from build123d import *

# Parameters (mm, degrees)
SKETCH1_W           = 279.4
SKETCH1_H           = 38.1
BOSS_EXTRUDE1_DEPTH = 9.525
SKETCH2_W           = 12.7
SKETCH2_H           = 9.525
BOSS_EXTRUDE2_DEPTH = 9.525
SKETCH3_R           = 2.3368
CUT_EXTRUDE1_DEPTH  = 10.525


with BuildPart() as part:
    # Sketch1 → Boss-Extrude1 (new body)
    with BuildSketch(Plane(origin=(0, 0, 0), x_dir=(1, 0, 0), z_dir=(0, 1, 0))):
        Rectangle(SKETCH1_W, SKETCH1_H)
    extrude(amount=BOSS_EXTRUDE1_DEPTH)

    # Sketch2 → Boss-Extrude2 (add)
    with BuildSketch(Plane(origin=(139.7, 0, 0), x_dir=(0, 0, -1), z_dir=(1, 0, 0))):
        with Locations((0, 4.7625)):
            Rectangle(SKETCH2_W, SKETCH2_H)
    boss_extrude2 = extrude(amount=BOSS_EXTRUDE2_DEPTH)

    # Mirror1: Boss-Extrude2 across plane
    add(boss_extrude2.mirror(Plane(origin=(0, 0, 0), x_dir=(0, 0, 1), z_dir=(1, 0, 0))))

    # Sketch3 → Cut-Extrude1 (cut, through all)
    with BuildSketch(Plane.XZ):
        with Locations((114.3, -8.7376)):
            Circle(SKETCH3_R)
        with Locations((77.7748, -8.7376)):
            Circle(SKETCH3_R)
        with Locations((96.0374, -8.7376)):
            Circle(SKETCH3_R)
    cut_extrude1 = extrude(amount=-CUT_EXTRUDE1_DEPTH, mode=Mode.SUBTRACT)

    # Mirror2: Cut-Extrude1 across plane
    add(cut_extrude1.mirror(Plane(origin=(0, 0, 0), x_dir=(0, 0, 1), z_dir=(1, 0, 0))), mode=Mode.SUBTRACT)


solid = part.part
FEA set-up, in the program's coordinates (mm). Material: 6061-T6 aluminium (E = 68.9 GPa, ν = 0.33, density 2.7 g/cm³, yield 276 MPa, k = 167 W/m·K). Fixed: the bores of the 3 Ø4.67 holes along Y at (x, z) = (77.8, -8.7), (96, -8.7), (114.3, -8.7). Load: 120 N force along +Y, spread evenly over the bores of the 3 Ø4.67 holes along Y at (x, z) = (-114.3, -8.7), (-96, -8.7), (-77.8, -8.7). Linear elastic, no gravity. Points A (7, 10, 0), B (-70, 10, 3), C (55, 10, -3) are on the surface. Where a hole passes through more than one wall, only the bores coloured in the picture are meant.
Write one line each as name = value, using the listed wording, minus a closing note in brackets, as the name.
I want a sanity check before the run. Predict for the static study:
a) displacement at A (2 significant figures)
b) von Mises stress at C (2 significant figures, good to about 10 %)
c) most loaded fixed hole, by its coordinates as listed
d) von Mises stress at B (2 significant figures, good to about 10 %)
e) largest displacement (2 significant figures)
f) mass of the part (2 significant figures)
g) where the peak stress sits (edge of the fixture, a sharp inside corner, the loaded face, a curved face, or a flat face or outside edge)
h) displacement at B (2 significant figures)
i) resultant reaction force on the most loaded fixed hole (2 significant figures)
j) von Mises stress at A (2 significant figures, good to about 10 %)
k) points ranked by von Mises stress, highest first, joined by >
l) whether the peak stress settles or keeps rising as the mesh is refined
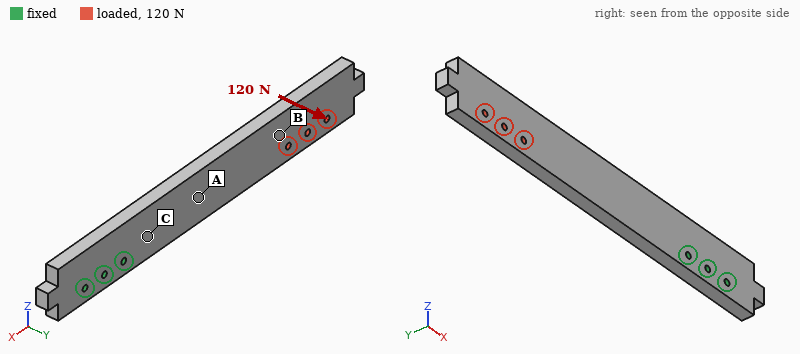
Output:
displacement at A = 0.26 mm
von Mises stress at C = 31 MPa
most loaded fixed hole, by its coordinates as listed = (77.8, -8.7)
von Mises stress at B = 5.9 MPa
largest displacement = 1.7 mm
mass of the part = 280 g
where the peak stress sits = edge of the fixture
displacement at B = 0.91 mm
resultant reaction force on the most loaded fixed hole = 590 N
von Mises stress at A = 22 MPa
points ranked by von Mises stress, highest first, joined by > = C > A > B
whether the peak stress settles or keeps rising as the mesh is refined = keeps rising
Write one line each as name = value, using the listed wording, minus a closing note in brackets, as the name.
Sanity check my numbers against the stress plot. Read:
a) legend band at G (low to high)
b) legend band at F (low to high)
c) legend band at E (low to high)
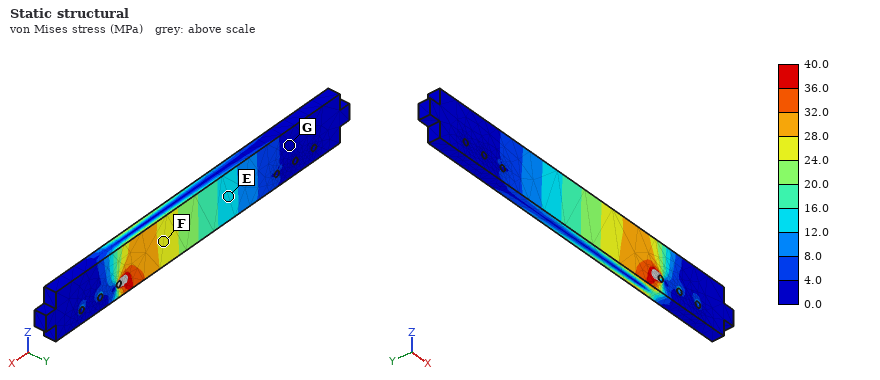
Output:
legend band at G = 0.0 to 4.0 MPa
legend band at F = 24.0 to 28.0 MPa
legend band at E = 12.0 to 16.0 MPa
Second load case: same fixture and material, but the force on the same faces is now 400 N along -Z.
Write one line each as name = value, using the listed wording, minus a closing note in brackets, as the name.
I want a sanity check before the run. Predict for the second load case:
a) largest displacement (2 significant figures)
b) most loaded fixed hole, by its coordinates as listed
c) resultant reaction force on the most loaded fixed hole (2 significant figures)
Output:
largest displacement = 0.45 mm
most loaded fixed hole, by its coordinates as listed = (77.8, -8.7)
resultant reaction force on the most loaded fixed hole = 2.7 kN
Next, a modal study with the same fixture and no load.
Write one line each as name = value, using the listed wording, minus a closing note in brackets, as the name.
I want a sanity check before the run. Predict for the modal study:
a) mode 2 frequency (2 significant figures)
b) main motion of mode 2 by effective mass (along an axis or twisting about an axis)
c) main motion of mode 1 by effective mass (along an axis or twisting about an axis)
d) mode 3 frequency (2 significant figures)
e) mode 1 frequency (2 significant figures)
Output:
mode 2 frequency = 540 Hz
main motion of mode 2 by effective mass = along Z
main motion of mode 1 by effective mass = along Y
mode 3 frequency = 960 Hz
mode 1 frequency = 160 Hz
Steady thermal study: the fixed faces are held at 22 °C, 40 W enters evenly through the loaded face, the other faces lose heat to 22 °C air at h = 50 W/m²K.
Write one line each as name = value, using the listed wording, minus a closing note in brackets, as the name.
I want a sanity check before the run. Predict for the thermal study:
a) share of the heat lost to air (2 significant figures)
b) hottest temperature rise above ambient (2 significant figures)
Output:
share of the heat lost to air = 72 %
hottest temperature rise above ambient = 50 K
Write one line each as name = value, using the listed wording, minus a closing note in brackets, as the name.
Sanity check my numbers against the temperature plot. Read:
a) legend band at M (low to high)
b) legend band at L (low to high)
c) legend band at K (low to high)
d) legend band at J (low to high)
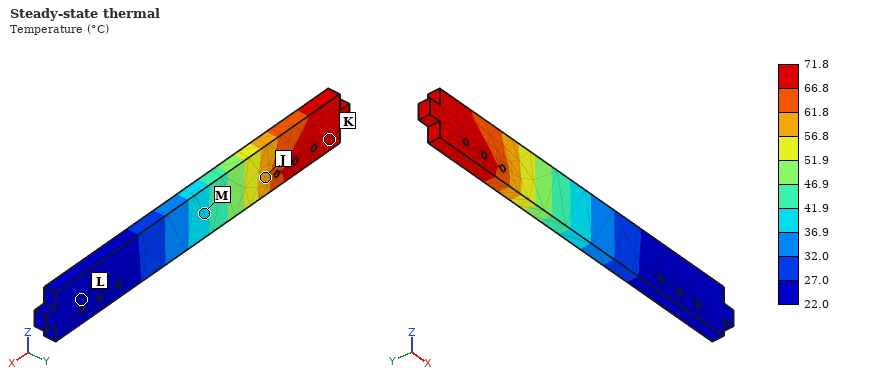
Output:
legend band at M = 36.9 to 41.9 °C
legend band at L = 22.0 to 27.0 °C
legend band at K = 66.8 to 71.8 °C
legend band at J = 56.8 to 61.8 °C
